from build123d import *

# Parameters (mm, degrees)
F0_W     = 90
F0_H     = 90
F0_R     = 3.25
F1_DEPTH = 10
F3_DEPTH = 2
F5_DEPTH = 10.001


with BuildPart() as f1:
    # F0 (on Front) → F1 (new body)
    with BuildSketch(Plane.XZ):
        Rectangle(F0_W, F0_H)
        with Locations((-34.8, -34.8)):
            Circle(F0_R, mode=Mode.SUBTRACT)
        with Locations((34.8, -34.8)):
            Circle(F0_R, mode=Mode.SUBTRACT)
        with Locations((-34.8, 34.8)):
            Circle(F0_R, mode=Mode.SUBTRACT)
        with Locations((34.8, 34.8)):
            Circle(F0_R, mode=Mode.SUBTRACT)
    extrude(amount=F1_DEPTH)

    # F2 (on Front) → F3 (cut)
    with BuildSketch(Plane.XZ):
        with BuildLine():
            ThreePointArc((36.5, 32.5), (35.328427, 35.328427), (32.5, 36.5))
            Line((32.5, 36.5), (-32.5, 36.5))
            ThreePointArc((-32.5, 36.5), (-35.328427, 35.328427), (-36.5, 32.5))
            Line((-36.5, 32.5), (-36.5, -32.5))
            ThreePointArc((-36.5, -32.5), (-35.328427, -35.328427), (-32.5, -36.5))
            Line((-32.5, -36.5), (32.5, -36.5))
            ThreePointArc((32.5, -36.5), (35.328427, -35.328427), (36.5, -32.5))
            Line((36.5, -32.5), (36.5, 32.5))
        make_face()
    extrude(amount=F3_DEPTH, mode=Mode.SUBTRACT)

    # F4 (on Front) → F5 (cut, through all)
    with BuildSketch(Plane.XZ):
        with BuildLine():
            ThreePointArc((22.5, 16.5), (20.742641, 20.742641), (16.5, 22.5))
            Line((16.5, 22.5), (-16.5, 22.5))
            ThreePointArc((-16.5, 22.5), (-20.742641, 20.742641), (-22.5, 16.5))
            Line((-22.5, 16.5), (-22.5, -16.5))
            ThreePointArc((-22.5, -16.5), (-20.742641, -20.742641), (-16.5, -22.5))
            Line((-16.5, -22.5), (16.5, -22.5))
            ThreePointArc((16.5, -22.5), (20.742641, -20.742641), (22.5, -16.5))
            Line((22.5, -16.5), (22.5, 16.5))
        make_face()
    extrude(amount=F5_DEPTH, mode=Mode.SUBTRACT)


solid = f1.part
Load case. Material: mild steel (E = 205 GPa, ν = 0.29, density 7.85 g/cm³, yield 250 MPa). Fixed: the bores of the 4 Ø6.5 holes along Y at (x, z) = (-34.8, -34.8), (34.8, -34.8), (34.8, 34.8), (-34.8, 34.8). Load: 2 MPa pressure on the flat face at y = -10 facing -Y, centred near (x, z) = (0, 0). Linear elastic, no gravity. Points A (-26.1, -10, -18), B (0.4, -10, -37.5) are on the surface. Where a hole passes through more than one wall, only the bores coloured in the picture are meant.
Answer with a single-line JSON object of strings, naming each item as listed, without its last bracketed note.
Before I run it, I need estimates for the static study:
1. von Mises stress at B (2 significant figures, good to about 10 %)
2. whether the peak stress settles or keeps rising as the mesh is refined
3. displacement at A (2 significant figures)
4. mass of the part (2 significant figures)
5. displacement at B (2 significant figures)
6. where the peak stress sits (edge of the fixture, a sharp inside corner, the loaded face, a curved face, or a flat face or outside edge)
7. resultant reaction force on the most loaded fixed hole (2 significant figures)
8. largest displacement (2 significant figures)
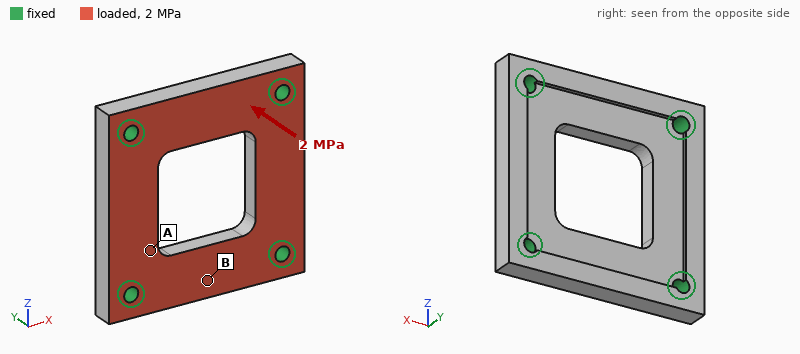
{"von Mises stress at B": "28 MPa", "whether the peak stress settles or keeps rising as the mesh is refined": "keeps rising", "displacement at A": "10 µm", "mass of the part": "420 g", "displacement at B": "11 µm", "where the peak stress sits": "edge of the fixture", "resultant reaction force on the most loaded fixed hole": "3.0 kN", "largest displacement": "17 µm"}
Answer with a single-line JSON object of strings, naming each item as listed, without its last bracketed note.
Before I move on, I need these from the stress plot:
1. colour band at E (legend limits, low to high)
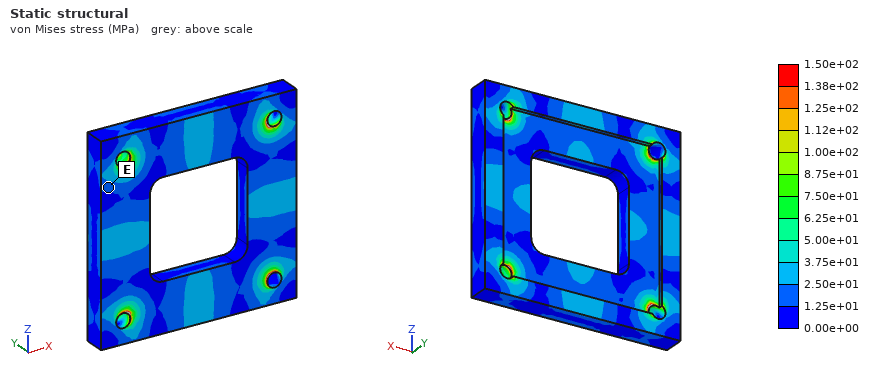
{"colour band at E": "1.25e+01 to 2.50e+01 MPa"}
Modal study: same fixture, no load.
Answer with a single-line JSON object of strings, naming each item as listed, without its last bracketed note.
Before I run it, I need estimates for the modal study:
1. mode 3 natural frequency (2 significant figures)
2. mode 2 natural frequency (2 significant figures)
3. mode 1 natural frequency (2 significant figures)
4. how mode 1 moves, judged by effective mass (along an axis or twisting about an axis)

{"mode 3 natural frequency": "9400 Hz", "mode 2 natural frequency": "9400 Hz", "mode 1 natural frequency": "8500 Hz", "how mode 1 moves, judged by effective mass": "along Y"}
